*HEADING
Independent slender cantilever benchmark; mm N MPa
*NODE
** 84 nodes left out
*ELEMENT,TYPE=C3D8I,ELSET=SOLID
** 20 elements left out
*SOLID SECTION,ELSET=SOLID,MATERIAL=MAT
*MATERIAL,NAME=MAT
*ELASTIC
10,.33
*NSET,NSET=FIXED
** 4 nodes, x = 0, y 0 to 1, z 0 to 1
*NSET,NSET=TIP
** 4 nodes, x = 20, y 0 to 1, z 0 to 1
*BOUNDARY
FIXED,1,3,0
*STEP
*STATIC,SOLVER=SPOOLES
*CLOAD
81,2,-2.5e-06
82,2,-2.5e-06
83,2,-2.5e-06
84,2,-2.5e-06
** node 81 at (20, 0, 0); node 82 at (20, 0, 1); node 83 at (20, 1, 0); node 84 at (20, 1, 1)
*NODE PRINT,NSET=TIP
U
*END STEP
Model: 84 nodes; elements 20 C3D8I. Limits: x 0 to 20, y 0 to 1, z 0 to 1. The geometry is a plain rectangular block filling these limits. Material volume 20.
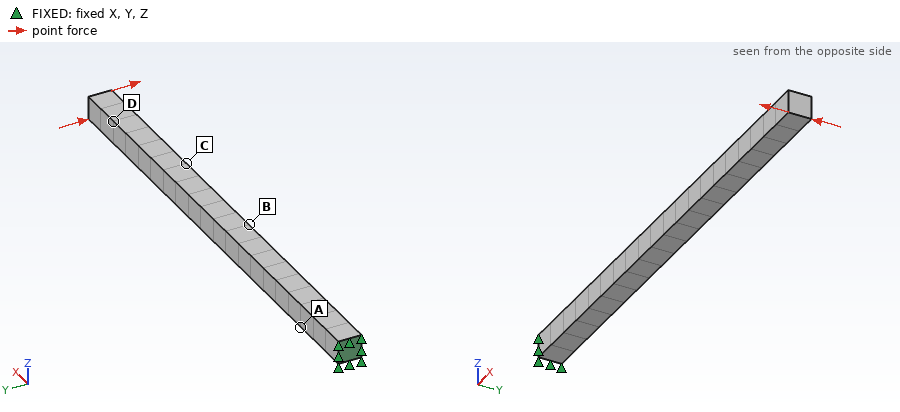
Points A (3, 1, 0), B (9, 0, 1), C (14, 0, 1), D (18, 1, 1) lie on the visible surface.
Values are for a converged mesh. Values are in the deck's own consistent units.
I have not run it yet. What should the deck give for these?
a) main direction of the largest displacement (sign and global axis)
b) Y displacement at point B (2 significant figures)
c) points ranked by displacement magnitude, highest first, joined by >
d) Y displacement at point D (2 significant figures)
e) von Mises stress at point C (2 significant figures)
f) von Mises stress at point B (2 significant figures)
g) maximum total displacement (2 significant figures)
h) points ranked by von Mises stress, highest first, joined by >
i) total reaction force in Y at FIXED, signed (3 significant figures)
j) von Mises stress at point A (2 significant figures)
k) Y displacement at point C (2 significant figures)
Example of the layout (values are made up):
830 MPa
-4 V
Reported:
-Y
-0.0081
D > C > B > A
-0.027
3.6e-04
6.6e-04
0.032
A > B > C > D
1.00e-05
0.0010
-0.018
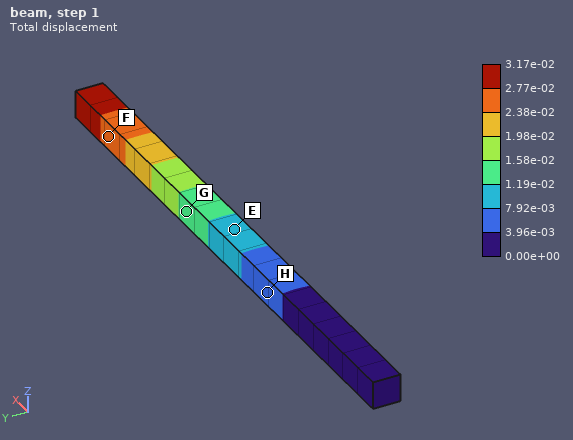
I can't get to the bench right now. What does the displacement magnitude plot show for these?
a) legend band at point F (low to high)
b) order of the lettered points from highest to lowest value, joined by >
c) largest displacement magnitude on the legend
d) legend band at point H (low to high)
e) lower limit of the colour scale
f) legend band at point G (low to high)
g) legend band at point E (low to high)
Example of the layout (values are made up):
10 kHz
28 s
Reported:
2.38e-02 to 2.77e-02
F > G > E > H
3.17e-02
3.96e-03 to 7.92e-03
0.00e+00
1.19e-02 to 1.58e-02
7.92e-03 to 1.19e-02
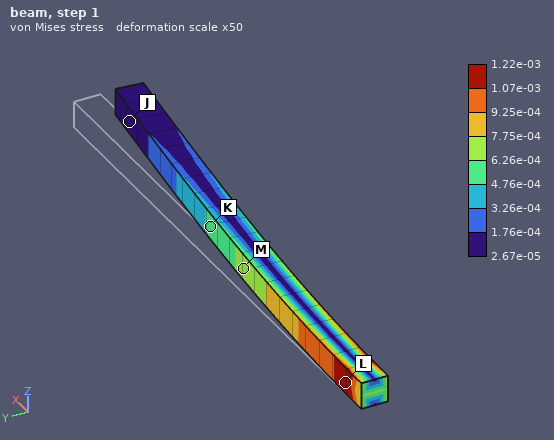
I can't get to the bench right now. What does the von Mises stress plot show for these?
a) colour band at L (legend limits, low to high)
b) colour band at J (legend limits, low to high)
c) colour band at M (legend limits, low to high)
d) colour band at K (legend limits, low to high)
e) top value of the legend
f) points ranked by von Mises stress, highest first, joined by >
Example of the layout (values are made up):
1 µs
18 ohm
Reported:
1.07e-03 to 1.22e-03
2.67e-05 to 1.76e-04
6.26e-04 to 7.75e-04
4.76e-04 to 6.26e-04
1.22e-03
L > M > K > J
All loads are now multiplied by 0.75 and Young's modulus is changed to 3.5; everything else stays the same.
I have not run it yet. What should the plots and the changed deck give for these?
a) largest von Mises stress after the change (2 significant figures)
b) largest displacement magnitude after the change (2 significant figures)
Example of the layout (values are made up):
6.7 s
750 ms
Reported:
9.2e-04
0.068
